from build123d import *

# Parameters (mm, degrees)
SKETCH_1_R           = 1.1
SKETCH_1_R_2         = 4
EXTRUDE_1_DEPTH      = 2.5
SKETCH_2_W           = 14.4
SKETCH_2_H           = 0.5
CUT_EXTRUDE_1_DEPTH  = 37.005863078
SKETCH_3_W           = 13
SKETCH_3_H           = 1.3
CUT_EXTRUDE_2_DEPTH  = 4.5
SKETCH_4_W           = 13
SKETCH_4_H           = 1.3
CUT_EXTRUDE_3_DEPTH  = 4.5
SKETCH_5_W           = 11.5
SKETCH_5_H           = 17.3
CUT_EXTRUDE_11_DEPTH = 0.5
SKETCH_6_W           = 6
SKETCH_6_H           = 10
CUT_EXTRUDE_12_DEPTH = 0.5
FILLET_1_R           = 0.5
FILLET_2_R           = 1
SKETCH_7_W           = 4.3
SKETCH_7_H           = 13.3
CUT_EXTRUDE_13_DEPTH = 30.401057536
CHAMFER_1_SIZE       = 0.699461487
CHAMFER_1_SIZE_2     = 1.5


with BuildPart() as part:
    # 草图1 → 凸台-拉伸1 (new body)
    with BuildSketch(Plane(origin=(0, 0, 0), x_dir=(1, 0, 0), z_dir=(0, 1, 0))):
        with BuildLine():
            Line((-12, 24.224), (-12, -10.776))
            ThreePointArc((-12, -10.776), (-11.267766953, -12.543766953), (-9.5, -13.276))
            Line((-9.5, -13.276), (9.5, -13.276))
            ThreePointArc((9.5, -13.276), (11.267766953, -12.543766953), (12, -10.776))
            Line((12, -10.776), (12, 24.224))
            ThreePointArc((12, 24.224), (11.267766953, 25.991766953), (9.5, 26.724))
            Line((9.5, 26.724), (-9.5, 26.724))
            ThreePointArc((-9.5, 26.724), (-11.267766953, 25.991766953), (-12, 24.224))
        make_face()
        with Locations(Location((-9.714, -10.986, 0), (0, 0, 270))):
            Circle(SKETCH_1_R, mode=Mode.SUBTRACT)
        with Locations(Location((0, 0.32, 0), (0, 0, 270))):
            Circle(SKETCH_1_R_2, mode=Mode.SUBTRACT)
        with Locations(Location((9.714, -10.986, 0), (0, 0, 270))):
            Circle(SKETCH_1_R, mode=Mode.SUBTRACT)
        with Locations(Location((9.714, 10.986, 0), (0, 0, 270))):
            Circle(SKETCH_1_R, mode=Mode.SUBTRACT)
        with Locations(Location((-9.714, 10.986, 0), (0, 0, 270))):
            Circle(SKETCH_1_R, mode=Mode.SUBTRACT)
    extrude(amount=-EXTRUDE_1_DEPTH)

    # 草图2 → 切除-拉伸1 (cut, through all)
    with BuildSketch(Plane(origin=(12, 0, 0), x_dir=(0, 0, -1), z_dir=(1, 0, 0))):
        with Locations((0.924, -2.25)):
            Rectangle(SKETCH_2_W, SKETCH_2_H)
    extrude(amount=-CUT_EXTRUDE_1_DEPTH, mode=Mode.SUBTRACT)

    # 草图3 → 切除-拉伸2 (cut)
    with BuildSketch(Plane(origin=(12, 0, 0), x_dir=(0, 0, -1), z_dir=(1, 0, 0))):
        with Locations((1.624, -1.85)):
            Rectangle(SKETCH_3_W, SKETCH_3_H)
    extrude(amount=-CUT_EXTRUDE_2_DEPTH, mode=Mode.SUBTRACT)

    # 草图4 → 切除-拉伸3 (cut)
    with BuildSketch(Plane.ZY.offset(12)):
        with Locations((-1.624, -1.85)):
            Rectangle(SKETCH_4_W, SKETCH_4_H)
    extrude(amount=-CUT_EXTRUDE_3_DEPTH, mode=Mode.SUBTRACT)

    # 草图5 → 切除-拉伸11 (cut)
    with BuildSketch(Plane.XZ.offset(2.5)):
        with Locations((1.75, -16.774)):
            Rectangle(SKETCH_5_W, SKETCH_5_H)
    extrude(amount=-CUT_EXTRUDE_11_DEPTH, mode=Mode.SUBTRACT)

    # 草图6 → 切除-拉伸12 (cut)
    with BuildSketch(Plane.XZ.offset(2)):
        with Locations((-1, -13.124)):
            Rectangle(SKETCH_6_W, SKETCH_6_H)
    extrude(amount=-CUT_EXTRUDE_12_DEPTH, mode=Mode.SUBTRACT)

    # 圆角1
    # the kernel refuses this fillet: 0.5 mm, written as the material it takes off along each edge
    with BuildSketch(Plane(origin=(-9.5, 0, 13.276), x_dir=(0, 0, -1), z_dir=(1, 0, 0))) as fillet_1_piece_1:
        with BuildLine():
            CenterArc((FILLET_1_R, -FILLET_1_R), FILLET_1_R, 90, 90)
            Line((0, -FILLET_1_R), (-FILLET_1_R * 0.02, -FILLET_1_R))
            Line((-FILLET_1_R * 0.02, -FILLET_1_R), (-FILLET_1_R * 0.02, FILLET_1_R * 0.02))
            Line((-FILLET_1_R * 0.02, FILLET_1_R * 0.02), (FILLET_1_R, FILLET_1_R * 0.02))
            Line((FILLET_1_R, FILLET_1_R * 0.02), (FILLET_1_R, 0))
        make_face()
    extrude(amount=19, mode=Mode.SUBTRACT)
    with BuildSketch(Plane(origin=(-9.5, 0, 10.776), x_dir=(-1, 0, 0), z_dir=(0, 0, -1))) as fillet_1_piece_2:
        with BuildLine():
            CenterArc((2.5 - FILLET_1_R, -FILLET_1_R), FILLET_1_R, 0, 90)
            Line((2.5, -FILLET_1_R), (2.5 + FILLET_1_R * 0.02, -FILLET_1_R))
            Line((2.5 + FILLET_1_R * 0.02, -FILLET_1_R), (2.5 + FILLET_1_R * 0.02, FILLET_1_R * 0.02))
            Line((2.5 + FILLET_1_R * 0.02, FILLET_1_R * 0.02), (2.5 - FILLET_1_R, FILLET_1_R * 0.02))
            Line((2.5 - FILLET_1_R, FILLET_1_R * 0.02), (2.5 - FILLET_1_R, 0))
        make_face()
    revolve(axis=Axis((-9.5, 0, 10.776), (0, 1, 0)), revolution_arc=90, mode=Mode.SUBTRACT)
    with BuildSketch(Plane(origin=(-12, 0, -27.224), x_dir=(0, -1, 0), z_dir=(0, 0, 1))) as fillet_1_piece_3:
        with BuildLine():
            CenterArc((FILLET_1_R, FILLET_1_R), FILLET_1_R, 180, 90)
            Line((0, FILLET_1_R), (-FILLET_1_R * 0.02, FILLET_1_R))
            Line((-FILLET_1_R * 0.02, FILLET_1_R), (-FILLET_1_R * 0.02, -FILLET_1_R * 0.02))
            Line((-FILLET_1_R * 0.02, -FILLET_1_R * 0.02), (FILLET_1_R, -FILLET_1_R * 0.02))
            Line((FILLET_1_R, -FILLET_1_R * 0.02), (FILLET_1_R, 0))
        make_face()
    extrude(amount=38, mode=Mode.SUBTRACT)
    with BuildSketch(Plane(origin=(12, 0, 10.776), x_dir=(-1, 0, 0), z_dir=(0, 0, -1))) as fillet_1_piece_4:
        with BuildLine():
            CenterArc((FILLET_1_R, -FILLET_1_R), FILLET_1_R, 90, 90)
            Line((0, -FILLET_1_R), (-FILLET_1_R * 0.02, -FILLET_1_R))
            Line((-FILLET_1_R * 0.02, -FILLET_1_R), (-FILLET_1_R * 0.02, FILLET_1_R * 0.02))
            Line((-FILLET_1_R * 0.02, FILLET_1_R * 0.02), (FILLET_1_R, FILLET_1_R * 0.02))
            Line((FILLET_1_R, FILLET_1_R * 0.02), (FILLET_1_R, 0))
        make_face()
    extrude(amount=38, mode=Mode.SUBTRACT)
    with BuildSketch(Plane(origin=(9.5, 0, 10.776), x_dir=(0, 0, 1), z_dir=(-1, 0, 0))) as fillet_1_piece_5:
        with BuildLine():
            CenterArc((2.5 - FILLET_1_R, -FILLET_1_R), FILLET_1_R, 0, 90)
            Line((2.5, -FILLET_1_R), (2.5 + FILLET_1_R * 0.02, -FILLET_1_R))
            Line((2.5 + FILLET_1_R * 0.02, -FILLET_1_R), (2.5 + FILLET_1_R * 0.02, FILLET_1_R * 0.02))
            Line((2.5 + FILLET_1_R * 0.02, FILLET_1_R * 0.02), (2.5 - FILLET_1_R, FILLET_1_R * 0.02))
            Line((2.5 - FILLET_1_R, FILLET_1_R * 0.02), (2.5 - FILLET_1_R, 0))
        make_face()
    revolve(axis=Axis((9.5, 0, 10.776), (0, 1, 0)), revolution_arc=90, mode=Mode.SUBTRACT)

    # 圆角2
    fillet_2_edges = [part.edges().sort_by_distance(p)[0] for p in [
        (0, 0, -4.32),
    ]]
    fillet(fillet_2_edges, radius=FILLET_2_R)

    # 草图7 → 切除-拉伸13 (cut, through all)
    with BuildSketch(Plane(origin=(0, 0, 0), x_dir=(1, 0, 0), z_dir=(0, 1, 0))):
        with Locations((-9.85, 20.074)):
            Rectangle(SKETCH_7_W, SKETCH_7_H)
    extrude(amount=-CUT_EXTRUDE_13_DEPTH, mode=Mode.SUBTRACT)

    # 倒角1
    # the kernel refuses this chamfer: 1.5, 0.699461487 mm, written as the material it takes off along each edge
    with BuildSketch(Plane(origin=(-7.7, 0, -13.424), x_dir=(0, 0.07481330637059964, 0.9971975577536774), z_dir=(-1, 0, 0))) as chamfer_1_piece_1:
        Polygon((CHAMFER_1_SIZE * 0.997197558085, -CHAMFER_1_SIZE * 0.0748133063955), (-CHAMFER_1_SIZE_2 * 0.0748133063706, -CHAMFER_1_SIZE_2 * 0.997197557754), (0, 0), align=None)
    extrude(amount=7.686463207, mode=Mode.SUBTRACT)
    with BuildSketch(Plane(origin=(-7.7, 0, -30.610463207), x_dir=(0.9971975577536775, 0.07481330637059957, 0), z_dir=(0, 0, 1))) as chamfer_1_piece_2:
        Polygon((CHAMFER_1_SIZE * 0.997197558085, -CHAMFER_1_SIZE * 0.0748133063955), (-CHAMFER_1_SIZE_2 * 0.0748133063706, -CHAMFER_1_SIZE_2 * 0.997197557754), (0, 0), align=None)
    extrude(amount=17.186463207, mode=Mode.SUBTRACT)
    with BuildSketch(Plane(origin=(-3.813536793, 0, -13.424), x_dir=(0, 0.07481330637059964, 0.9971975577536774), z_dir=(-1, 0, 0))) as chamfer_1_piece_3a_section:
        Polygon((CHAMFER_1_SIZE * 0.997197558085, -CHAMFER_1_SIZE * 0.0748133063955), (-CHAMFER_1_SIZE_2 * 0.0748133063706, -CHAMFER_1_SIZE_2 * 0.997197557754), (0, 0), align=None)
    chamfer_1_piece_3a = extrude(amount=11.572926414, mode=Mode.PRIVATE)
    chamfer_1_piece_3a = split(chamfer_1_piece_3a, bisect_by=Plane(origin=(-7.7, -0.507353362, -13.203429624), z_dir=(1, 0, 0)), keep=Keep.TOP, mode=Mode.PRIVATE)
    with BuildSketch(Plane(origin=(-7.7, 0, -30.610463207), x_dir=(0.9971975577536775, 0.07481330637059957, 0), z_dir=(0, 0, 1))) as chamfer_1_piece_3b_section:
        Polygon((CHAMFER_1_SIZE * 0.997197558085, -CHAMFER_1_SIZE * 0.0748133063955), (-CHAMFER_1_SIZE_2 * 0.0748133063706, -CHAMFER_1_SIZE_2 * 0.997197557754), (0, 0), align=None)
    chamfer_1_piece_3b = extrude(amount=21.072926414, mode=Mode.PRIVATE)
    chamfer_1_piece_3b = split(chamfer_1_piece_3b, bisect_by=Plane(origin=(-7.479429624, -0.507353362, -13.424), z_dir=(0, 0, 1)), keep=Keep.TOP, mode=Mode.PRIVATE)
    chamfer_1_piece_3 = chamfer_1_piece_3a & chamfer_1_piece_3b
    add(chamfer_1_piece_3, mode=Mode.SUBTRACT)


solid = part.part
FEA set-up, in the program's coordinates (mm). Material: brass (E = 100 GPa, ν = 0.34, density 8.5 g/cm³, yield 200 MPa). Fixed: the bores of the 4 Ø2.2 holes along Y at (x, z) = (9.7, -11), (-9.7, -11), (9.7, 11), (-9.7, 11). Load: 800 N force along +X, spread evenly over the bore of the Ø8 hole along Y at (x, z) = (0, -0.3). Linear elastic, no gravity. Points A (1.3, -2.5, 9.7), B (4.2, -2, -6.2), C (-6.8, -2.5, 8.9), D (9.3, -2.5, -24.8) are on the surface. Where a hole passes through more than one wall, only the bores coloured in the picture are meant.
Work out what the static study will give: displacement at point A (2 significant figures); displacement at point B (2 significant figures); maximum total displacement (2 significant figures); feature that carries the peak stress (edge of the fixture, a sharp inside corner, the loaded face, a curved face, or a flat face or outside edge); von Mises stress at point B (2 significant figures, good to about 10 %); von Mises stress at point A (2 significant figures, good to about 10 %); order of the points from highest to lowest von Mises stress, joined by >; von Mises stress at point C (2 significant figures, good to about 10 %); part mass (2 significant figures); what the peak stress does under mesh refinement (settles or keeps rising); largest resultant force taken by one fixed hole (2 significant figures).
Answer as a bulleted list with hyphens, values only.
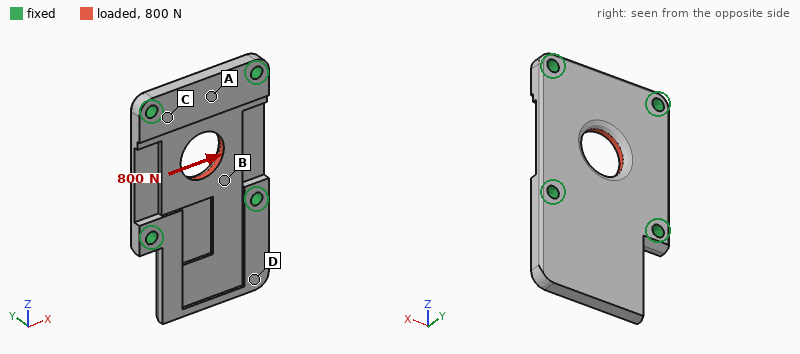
- 0.79 µm
- 1.9 µm
- 4.0 µm
- edge of the fixture
- 22 MPa
- 10 MPa
- B > C > A > D
- 18 MPa
- 14 g
- keeps rising
- 240 N
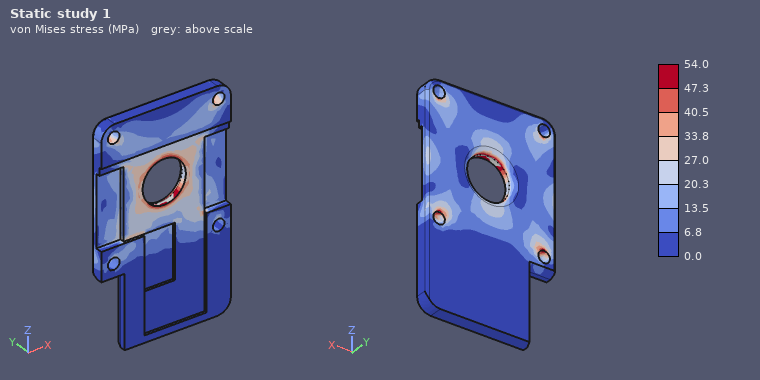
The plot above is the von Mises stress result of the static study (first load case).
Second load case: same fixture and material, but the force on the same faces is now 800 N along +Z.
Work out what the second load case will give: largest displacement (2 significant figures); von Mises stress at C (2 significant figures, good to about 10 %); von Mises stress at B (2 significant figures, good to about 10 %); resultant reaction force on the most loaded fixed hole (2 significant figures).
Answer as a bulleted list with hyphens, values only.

- 3.4 µm
- 13 MPa
- 22 MPa
- 220 N
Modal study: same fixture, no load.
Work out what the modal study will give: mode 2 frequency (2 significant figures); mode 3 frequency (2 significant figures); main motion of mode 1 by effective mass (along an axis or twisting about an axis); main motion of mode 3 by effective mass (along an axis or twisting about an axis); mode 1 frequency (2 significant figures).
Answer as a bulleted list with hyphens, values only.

- 9600 Hz
- 13 kHz
- along Y
- along Y
- 4400 Hz
